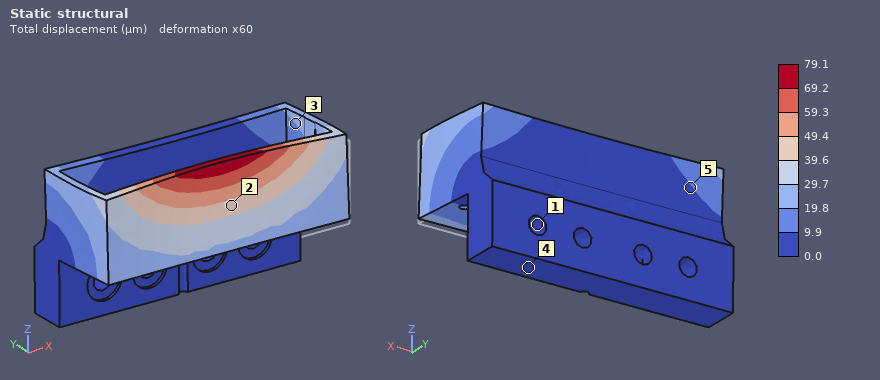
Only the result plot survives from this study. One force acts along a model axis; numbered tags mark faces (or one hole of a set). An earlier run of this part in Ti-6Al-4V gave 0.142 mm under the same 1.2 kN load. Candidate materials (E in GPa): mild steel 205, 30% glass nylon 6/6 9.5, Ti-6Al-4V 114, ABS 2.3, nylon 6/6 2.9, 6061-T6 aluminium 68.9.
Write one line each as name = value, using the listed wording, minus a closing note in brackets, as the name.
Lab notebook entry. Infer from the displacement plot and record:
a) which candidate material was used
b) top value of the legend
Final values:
which candidate material was used = mild steel
top value of the legend = 79.1 µm
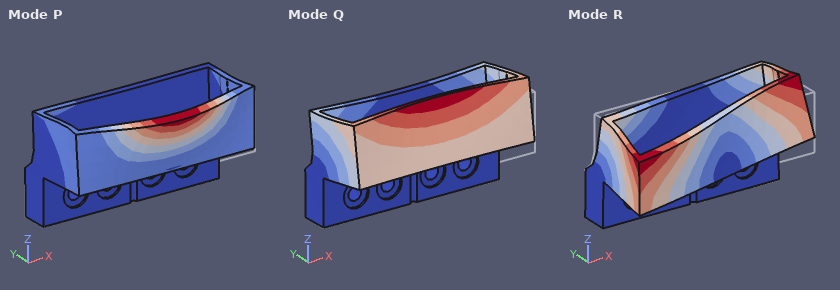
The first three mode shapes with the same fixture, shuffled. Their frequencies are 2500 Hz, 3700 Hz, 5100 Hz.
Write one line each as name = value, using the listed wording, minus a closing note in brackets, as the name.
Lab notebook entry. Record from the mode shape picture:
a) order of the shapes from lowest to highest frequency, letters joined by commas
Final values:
order of the shapes from lowest to highest frequency, letters joined by commas = Q, R, P
